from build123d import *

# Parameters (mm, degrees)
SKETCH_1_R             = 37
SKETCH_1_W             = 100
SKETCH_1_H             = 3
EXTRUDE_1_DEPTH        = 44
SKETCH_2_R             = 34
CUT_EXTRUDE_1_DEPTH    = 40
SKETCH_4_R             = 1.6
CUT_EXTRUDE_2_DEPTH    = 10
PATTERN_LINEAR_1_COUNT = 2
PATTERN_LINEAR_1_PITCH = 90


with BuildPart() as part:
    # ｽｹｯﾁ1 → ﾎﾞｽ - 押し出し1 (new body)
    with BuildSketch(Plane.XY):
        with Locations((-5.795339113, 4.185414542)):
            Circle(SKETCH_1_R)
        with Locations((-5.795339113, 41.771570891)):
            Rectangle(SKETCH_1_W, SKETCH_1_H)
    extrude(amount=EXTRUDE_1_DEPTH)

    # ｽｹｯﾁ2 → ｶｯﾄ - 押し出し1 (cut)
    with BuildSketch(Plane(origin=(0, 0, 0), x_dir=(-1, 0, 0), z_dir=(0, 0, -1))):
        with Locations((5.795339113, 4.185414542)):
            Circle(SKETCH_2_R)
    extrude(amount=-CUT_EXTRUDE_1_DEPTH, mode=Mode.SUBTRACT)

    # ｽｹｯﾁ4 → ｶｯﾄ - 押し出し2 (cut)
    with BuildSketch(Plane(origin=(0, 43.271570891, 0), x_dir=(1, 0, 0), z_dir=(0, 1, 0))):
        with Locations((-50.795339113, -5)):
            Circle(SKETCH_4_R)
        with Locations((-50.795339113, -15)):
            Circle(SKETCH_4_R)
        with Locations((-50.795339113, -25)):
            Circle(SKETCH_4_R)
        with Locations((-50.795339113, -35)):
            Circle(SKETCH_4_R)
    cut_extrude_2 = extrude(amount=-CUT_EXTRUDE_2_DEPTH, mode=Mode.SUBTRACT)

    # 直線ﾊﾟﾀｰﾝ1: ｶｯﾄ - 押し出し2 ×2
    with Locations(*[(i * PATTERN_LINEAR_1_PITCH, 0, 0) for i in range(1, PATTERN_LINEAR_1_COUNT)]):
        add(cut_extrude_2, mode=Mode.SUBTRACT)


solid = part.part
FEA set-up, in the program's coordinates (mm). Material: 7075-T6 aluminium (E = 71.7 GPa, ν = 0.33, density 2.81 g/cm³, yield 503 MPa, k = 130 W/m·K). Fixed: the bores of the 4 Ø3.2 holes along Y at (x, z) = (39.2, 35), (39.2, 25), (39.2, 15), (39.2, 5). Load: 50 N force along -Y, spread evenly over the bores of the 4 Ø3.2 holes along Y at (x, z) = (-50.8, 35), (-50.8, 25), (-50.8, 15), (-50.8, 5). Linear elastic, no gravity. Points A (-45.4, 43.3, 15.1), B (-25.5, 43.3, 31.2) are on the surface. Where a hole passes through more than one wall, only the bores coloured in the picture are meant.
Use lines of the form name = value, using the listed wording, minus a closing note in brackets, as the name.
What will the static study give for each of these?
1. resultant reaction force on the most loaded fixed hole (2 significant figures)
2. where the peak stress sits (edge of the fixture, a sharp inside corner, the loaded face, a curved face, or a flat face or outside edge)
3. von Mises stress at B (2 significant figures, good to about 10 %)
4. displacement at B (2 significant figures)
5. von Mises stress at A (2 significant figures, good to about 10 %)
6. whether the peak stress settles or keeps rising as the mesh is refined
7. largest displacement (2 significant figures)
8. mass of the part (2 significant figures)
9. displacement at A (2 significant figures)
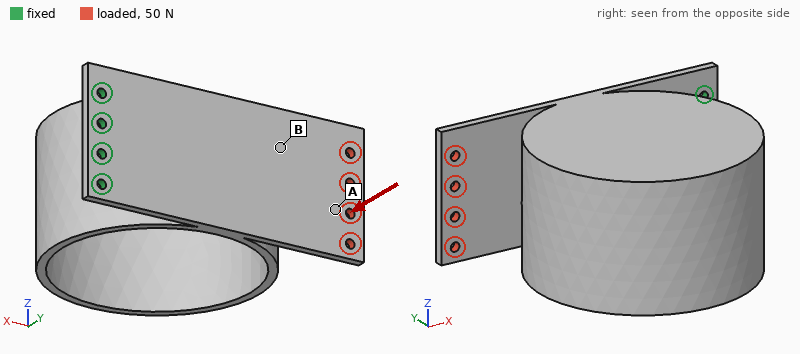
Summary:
resultant reaction force on the most loaded fixed hole = 38 N
where the peak stress sits = edge of the fixture
von Mises stress at B = 17 MPa
displacement at B = 0.85 mm
von Mises stress at A = 4.9 MPa
whether the peak stress settles or keeps rising as the mesh is refined = keeps rising
largest displacement = 1.5 mm
mass of the part = 160 g
displacement at A = 1.3 mm
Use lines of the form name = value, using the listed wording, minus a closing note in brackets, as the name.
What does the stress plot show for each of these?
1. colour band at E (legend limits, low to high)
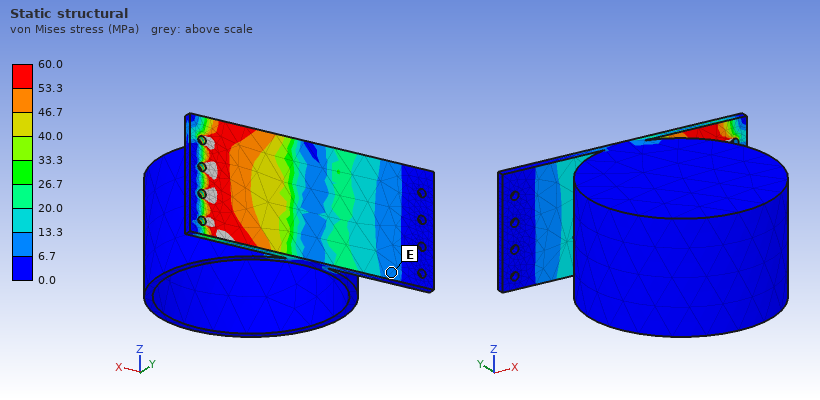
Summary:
colour band at E = 6.7 to 13.3 MPa
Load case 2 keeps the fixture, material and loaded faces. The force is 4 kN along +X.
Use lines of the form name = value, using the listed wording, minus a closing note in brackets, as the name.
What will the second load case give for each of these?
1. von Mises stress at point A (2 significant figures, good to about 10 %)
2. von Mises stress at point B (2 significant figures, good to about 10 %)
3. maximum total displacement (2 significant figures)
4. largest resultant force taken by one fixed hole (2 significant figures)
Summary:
von Mises stress at point A = 36 MPa
von Mises stress at point B = 29 MPa
maximum total displacement = 96 µm
largest resultant force taken by one fixed hole = 1.1 kN
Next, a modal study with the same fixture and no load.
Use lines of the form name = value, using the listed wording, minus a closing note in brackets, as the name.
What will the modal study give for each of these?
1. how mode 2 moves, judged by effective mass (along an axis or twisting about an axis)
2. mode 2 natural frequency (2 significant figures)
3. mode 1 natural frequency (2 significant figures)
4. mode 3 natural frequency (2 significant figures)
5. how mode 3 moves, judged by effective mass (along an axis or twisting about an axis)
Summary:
how mode 2 moves, judged by effective mass = along Z
mode 2 natural frequency = 220 Hz
mode 1 natural frequency = 110 Hz
mode 3 natural frequency = 550 Hz
how mode 3 moves, judged by effective mass = along Y
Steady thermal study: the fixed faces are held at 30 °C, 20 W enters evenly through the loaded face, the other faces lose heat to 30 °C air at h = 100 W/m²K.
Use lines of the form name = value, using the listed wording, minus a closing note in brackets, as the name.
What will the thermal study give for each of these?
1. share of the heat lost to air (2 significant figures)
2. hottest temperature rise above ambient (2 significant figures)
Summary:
share of the heat lost to air = 90 %
hottest temperature rise above ambient = 41 K
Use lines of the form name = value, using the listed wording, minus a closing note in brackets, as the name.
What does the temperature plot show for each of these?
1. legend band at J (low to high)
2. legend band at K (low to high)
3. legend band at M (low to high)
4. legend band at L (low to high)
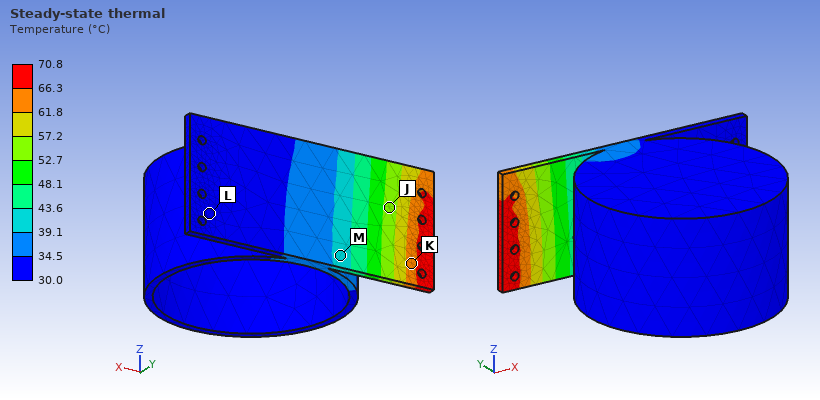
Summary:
legend band at J = 52.7 to 57.2 °C
legend band at K = 61.8 to 66.3 °C
legend band at M = 39.1 to 43.6 °C
legend band at L = 30.0 to 34.5 °C
